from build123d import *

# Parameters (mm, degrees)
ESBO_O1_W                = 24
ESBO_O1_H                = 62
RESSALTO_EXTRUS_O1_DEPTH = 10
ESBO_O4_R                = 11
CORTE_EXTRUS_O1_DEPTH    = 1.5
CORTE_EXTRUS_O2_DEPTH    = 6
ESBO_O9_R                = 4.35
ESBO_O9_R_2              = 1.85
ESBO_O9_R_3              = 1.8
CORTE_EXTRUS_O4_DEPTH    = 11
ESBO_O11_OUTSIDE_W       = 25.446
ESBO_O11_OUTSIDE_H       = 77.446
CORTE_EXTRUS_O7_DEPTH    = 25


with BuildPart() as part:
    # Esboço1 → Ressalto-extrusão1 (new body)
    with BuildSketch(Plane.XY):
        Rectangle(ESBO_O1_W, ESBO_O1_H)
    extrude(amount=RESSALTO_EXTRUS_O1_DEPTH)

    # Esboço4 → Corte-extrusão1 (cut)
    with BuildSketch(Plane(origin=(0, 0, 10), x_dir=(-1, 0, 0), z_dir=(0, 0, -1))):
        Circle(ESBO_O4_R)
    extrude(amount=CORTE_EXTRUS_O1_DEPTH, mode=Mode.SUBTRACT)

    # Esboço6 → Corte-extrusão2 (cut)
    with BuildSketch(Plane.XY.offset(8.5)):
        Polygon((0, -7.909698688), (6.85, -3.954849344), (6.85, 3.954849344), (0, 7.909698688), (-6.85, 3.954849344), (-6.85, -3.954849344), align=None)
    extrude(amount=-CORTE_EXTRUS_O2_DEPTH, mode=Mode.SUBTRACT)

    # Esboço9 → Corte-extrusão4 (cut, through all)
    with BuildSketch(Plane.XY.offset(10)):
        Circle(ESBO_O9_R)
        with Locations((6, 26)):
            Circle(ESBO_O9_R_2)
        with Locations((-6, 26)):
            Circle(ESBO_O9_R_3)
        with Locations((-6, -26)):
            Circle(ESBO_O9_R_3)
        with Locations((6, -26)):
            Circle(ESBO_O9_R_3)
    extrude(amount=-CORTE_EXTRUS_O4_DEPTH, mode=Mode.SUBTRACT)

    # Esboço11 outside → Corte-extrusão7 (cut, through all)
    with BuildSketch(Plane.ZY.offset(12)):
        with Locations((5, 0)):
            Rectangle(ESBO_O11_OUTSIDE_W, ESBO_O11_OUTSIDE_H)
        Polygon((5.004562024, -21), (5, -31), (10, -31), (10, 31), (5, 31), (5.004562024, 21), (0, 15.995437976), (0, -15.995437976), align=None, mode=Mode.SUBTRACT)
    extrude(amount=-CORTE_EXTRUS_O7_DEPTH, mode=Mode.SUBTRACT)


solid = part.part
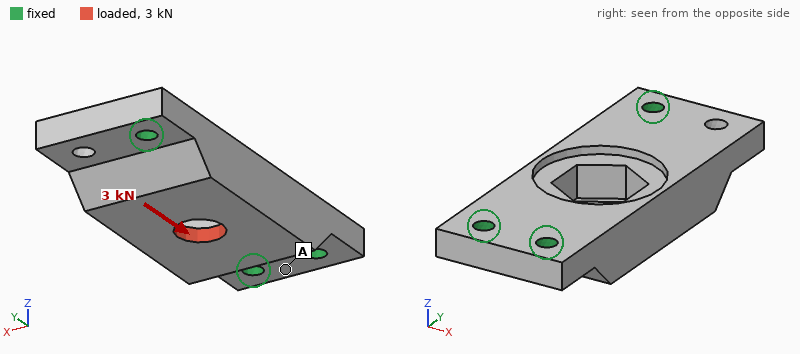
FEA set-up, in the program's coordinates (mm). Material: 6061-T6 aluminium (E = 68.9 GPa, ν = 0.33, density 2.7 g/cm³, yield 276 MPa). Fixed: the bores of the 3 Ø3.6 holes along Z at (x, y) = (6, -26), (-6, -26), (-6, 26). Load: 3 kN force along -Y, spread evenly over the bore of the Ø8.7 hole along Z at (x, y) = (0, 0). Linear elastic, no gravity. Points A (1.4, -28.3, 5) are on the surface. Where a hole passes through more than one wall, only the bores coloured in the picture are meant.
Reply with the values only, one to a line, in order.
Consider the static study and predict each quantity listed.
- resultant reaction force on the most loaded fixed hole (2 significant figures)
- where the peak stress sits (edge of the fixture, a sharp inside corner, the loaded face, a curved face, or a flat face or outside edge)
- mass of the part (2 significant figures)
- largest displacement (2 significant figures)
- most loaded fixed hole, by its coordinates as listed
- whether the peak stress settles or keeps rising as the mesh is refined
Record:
1.3 kN
edge of the fixture
27 g
12 µm
(-6, 26)
keeps rising
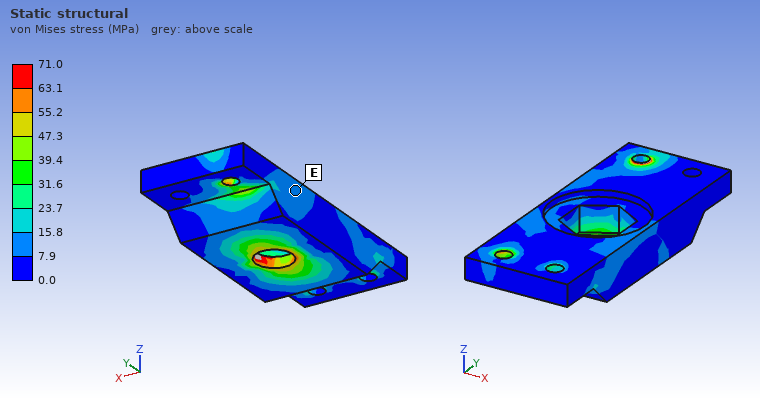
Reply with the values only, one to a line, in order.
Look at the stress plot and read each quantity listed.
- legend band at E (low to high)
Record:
7.9 to 15.8 MPa
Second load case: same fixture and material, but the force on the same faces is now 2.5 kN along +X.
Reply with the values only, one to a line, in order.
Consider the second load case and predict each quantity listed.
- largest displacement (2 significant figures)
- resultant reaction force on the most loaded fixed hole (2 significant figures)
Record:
45 µm
1.7 kN
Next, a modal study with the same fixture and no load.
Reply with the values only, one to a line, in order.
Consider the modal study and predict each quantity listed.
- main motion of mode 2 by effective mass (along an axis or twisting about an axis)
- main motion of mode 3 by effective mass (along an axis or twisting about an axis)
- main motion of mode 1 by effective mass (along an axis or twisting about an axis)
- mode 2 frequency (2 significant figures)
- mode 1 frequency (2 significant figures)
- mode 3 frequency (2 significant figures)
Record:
along Z
along X
along Z
13 kHz
9000 Hz
18 kHz
